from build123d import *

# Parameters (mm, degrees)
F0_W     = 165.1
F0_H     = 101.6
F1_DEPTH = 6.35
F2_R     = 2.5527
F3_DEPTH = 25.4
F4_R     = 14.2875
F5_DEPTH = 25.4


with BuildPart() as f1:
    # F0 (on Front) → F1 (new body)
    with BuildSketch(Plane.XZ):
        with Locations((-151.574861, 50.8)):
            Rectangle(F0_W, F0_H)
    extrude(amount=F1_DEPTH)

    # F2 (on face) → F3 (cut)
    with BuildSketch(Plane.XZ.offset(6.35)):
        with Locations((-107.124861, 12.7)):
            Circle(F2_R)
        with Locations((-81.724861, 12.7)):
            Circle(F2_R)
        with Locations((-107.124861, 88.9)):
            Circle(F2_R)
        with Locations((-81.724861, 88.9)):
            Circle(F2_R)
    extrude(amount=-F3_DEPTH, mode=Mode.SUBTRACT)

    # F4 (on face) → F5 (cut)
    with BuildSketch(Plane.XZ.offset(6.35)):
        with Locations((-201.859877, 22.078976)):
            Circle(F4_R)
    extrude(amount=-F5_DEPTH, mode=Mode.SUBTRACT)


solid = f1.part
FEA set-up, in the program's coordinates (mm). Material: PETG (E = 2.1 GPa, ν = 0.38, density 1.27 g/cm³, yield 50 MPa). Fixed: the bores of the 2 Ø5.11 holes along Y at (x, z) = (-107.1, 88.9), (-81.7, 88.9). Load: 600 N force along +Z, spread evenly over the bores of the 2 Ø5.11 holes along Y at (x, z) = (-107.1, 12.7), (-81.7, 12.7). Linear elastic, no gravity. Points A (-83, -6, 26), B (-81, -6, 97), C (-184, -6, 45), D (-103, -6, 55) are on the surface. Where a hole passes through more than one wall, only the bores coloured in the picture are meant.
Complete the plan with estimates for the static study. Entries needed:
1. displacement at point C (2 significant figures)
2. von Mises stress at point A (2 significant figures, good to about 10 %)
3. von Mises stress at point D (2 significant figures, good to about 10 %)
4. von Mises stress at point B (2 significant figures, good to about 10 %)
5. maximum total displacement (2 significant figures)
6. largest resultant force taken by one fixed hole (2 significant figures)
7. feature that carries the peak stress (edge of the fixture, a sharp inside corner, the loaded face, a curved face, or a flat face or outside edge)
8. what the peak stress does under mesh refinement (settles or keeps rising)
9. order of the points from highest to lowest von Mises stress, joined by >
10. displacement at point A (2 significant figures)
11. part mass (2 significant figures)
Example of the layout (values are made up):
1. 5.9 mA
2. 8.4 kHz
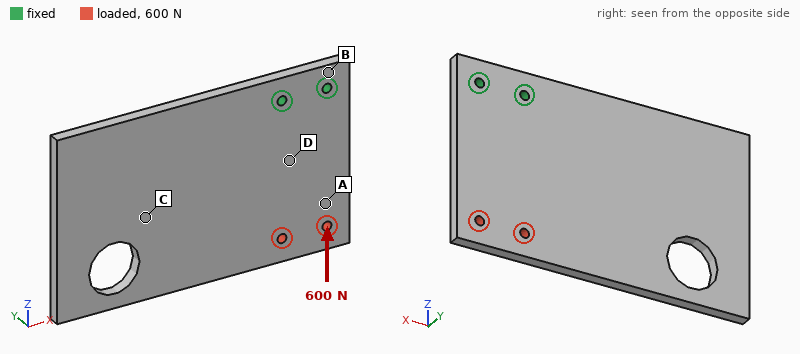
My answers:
1. 17 µm
2. 2.2 MPa
3. 1.6 MPa
4. 0.78 MPa
5. 85 µm
6. 300 N
7. edge of the fixture
8. keeps rising
9. A > D > B > C
10. 64 µm
11. 130 g
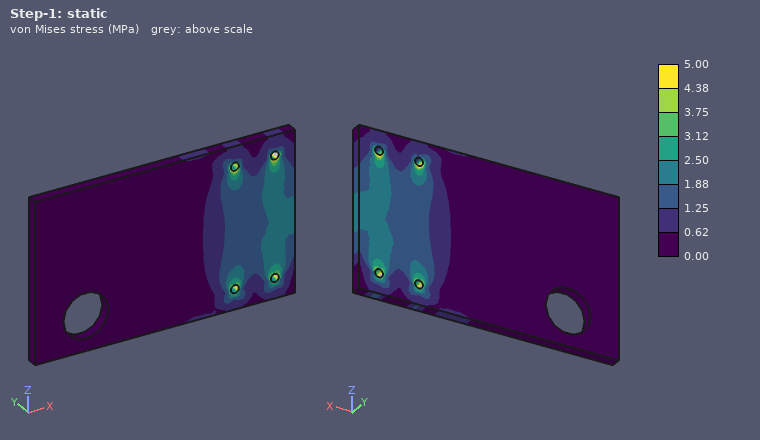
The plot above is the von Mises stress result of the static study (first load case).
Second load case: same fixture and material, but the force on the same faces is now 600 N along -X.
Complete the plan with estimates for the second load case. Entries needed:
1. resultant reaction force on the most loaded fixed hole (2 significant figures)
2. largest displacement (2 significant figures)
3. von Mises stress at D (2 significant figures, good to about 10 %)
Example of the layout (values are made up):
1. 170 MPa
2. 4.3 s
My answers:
1. 1.6 kN
2. 1.8 mm
3. 4.7 MPa
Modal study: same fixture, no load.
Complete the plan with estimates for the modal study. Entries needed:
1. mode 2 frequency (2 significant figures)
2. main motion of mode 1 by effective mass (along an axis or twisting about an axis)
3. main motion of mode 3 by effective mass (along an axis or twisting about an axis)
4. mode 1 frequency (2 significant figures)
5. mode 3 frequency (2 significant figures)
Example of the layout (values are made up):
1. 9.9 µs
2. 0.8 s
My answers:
1. 130 Hz
2. along Y
3. along Y
4. 64 Hz
5. 280 Hz
